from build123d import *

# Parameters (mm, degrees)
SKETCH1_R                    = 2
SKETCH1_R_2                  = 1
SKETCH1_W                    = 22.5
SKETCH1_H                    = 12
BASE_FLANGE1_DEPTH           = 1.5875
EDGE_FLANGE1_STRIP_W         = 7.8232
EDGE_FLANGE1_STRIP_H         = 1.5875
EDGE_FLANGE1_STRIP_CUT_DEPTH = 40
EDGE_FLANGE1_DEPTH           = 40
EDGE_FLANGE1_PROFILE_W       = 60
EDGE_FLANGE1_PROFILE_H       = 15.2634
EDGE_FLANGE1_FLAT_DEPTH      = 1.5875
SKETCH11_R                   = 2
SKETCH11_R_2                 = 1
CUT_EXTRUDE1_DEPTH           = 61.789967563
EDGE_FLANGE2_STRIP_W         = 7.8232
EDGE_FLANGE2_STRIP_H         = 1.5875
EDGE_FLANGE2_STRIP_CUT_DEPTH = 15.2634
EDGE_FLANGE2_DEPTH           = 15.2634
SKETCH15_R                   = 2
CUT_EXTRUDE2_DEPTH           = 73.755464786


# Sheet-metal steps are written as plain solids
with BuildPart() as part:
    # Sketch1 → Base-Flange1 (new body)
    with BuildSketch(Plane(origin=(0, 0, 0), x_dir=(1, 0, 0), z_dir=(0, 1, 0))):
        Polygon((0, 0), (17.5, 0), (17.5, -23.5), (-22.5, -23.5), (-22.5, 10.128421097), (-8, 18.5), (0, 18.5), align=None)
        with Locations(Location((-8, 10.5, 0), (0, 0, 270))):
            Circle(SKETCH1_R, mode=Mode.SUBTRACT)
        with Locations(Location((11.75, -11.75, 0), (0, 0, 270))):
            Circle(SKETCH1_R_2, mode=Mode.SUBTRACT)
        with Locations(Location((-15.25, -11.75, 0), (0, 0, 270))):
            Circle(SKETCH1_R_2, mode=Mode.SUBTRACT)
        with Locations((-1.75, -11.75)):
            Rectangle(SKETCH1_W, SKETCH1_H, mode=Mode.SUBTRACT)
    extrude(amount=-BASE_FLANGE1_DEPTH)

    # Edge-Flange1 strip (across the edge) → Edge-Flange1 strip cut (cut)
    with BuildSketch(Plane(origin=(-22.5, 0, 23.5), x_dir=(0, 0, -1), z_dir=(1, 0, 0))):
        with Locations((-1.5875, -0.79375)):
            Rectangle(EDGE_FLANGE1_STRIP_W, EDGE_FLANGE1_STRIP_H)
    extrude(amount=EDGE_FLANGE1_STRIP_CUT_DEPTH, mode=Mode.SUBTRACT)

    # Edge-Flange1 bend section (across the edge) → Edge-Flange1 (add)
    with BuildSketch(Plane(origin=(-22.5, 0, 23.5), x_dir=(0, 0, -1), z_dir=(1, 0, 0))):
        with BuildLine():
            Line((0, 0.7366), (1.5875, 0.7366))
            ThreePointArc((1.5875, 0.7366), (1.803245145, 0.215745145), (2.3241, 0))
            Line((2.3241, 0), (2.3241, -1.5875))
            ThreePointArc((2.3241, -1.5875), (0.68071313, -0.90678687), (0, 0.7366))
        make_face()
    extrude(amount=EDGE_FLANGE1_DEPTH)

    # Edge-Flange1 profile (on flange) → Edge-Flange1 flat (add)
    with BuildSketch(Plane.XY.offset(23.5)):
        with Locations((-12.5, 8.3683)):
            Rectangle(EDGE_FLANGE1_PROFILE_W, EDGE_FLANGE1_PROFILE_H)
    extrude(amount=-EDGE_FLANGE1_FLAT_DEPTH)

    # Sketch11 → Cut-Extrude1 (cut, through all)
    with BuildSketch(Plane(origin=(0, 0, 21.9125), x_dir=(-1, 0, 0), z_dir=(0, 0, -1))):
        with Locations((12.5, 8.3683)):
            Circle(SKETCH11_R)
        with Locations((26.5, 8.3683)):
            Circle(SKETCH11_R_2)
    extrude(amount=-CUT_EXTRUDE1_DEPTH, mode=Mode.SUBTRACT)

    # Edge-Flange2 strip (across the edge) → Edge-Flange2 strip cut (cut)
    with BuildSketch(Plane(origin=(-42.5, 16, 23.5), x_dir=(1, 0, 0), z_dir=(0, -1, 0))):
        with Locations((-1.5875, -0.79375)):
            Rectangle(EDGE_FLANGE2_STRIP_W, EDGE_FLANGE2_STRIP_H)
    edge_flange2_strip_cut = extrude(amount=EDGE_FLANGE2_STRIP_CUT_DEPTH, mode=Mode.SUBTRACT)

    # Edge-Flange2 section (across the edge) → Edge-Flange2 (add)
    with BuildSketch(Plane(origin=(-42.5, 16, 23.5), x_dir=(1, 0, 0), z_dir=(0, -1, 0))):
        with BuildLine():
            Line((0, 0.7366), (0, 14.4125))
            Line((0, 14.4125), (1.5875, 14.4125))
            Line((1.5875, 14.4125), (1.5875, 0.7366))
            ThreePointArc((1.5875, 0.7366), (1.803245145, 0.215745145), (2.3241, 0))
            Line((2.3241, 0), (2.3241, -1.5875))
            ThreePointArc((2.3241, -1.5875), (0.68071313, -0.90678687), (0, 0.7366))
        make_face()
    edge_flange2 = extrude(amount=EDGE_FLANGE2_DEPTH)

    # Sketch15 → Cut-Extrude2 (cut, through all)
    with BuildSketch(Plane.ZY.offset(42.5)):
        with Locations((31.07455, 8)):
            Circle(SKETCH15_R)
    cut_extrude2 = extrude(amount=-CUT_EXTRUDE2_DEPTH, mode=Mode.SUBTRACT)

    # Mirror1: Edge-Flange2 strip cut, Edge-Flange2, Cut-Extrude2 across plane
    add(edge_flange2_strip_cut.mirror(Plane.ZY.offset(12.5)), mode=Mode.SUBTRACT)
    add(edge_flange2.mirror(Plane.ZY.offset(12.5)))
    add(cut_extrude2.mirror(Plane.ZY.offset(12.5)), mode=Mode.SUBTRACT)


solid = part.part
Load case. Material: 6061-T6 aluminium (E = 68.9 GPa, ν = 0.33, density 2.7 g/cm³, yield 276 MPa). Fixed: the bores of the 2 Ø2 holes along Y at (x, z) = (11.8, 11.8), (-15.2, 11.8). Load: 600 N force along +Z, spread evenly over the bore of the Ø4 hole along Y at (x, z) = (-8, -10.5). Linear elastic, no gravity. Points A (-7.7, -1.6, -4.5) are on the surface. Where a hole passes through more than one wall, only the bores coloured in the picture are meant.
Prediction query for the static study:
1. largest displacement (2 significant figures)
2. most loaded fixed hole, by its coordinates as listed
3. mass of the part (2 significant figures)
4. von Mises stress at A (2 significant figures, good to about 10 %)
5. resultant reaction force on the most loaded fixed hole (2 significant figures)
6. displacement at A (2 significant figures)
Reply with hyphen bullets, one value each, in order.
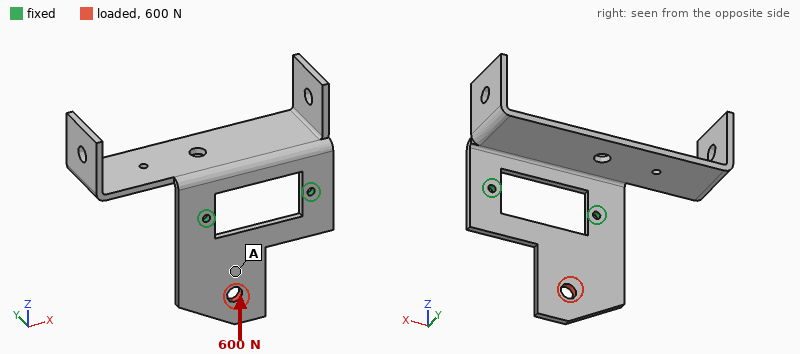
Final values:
- 46 µm
- (-15.2, 11.8)
- 9.9 g
- 20 MPa
- 460 N
- 24 µm
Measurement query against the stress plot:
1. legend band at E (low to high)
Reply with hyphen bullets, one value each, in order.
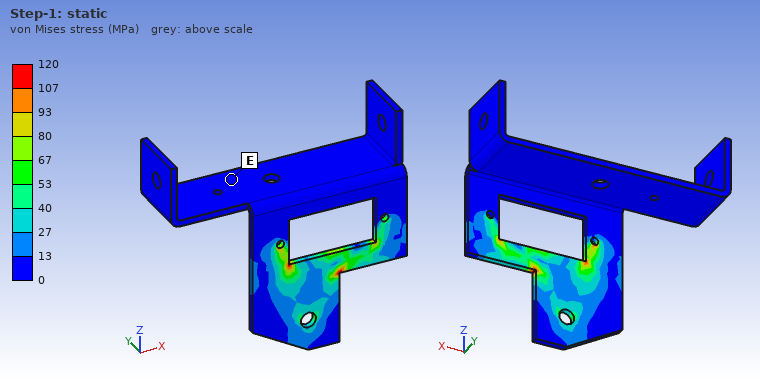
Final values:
- 0 to 13 MPa
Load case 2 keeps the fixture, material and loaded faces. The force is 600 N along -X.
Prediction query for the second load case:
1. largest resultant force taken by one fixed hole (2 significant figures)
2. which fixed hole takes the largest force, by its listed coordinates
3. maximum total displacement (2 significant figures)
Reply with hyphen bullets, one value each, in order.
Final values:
- 560 N
- (11.8, 11.8)
- 0.12 mm
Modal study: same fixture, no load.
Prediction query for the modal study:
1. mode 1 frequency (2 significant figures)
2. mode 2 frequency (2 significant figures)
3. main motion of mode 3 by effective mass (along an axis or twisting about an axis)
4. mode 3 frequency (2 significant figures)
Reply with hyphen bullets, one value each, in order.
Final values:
- 770 Hz
- 1100 Hz
- along Y
- 1400 Hz
